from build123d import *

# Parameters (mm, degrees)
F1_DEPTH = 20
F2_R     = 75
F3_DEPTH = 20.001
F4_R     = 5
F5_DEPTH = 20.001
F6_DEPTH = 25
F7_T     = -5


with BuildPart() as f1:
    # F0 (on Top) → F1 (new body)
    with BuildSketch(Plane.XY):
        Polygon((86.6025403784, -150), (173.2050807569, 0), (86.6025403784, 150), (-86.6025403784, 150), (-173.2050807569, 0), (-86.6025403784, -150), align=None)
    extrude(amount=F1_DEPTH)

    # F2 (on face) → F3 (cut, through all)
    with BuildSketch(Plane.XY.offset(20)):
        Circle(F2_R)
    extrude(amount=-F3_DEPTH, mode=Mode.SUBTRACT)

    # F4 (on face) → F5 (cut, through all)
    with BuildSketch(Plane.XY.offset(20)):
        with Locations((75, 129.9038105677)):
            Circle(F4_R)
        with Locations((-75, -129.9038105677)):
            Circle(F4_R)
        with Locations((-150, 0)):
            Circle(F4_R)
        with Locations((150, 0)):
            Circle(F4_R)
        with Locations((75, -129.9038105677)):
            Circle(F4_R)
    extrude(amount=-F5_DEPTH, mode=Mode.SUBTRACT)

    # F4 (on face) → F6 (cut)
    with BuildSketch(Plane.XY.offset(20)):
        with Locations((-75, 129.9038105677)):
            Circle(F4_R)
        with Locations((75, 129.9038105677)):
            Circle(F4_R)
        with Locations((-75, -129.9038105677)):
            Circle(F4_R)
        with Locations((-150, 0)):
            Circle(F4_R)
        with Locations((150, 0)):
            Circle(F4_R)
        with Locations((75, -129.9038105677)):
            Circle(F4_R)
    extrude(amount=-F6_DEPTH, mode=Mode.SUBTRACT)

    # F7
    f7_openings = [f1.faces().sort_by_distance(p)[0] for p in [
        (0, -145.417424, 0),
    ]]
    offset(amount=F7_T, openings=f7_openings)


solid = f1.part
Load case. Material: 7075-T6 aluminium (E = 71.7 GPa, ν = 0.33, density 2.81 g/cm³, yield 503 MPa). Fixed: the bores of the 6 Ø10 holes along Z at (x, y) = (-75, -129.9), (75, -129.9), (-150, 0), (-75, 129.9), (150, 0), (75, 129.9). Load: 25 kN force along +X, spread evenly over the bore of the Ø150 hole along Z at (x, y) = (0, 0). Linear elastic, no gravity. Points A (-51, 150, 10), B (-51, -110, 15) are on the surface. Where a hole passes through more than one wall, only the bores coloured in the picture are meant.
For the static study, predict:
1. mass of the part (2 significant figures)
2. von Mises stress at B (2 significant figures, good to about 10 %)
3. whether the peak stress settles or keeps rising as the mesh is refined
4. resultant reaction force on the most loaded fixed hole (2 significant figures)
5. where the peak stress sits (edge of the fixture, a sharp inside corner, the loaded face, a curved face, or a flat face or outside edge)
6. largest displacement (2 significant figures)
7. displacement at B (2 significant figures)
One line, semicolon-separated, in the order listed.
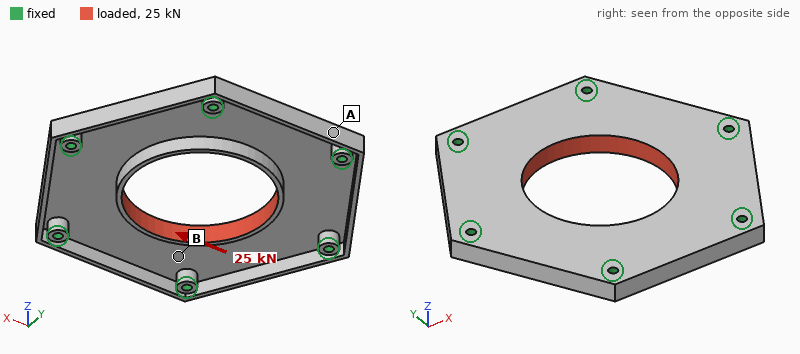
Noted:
1.2 kg; 20 MPa; keeps rising; 5.7 kN; edge of the fixture; 0.14 mm; 0.023 mm
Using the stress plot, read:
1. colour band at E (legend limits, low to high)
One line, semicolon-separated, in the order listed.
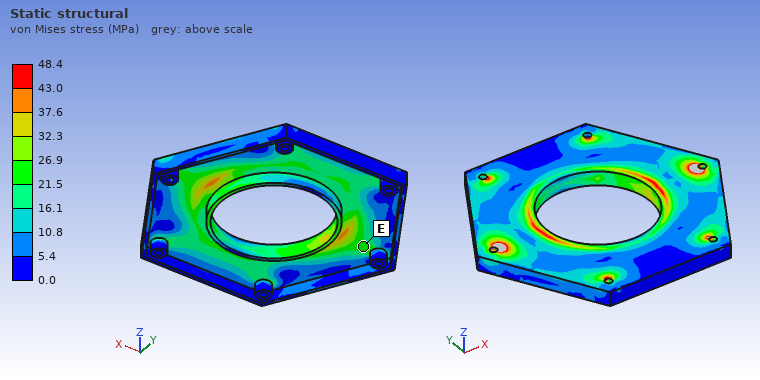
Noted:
21.5 to 26.9 MPa
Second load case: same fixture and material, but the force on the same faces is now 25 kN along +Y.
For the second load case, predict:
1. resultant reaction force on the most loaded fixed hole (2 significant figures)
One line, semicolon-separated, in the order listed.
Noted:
5.1 kN
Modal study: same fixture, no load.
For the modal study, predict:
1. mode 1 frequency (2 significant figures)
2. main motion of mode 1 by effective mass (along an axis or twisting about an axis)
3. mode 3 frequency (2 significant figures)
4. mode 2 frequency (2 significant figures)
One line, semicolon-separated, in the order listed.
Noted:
910 Hz; along Z; 1300 Hz; 1300 Hz
